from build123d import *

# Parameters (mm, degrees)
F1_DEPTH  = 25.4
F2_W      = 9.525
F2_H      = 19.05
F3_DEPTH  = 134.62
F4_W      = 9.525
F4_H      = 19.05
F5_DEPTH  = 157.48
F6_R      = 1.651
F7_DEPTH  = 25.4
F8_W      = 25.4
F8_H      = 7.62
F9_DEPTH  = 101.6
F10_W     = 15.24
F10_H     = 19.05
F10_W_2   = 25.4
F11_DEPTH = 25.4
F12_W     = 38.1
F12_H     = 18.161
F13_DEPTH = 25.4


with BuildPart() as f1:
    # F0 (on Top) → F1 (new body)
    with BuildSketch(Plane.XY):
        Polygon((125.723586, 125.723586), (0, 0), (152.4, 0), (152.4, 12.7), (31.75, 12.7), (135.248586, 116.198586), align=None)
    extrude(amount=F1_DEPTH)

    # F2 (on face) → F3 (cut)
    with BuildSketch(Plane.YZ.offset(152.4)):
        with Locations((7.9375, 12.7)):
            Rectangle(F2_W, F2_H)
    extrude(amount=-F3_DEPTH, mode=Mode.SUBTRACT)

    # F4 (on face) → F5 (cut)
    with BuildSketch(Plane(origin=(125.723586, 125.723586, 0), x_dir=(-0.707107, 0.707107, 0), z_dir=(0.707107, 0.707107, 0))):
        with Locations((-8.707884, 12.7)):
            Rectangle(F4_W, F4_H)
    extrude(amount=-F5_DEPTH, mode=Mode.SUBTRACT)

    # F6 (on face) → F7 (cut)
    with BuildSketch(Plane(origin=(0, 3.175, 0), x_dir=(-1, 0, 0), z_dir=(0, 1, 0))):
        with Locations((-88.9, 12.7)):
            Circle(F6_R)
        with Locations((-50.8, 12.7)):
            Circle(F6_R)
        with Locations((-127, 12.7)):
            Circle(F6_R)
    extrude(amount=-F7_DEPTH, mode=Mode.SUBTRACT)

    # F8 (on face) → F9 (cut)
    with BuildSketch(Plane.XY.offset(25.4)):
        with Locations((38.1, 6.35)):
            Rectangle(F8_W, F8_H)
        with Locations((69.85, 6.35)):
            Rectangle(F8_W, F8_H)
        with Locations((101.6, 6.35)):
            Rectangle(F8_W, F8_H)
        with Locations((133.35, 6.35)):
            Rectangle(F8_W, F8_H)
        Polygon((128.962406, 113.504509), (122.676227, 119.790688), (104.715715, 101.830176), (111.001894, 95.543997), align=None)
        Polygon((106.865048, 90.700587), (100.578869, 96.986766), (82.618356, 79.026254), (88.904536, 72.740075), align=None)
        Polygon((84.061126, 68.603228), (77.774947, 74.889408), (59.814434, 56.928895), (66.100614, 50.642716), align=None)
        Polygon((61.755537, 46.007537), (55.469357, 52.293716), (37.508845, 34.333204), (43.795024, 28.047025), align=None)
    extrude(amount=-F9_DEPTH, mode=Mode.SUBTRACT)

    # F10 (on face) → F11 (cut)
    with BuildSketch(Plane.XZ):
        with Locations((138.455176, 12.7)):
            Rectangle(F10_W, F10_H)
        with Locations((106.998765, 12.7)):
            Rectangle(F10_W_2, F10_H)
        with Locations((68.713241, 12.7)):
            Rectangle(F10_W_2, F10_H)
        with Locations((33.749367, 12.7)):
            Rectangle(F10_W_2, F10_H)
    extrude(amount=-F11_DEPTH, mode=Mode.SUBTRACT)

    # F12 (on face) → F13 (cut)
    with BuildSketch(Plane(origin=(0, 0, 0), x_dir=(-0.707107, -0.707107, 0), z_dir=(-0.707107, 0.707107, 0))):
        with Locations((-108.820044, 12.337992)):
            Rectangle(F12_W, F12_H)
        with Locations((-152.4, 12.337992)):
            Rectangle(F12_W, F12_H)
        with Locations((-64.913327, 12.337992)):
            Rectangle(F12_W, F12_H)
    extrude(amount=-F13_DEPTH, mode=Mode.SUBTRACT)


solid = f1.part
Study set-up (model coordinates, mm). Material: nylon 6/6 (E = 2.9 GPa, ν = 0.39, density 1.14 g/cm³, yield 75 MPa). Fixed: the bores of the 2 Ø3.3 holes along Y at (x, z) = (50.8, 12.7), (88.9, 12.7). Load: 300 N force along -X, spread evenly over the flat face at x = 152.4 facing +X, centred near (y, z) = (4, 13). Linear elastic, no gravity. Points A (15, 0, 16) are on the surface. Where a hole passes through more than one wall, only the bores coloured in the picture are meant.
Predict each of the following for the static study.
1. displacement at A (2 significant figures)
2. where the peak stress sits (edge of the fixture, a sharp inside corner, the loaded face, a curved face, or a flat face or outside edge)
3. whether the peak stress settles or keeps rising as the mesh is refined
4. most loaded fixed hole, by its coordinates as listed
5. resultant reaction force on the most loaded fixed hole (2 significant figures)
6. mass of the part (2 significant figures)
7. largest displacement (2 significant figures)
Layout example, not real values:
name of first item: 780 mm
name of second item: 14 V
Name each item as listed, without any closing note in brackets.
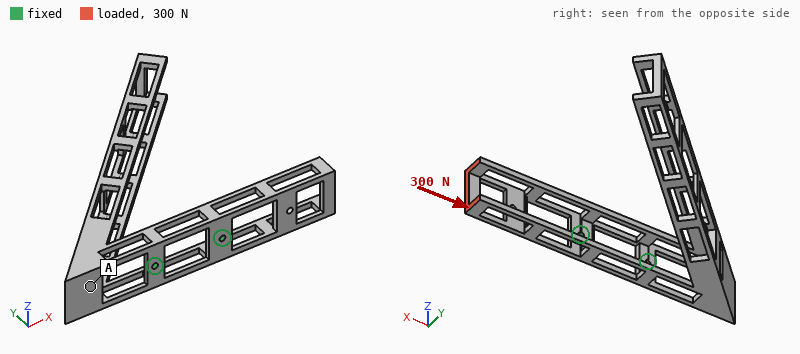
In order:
displacement at A: 0.52 mm
where the peak stress sits: edge of the fixture
whether the peak stress settles or keeps rising as the mesh is refined: keeps rising
most loaded fixed hole, by its coordinates as listed: (88.9, 12.7)
resultant reaction force on the most loaded fixed hole: 220 N
mass of the part: 25 g
largest displacement: 2.0 mm
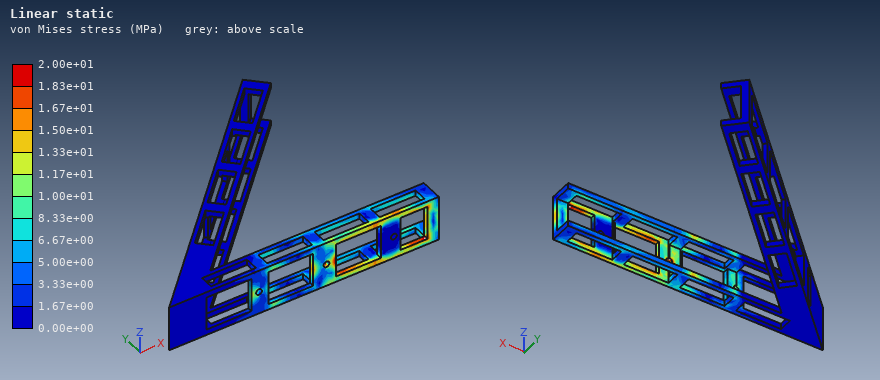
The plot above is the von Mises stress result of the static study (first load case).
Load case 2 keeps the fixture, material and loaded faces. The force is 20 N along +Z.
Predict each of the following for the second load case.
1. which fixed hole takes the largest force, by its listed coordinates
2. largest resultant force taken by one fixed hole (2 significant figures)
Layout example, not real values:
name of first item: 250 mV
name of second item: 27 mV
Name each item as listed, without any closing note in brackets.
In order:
which fixed hole takes the largest force, by its listed coordinates: (88.9, 12.7)
largest resultant force taken by one fixed hole: 27 N
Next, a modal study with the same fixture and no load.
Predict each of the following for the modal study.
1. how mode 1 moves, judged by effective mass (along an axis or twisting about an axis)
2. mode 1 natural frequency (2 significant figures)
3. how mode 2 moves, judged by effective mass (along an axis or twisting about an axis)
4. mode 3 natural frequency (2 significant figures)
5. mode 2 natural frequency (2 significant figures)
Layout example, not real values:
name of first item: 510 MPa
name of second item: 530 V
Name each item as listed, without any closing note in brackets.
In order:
how mode 1 moves, judged by effective mass: along Z
mode 1 natural frequency: 51 Hz
how mode 2 moves, judged by effective mass: along X
mode 3 natural frequency: 200 Hz
mode 2 natural frequency: 80 Hz
